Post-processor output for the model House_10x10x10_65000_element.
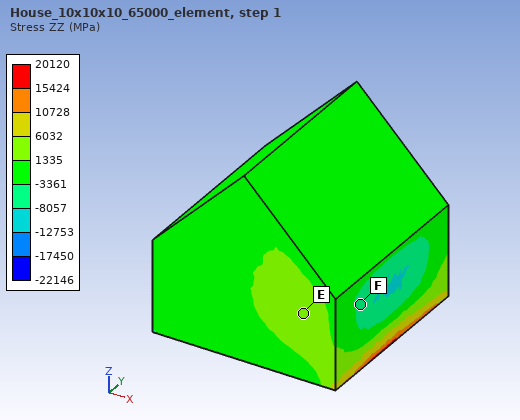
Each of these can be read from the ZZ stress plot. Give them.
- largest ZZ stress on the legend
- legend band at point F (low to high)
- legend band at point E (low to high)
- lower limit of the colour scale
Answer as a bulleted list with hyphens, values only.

- 20120 MPa
- -8057 to -3361 MPa
- 1335 to 6032 MPa
- -22146 MPa
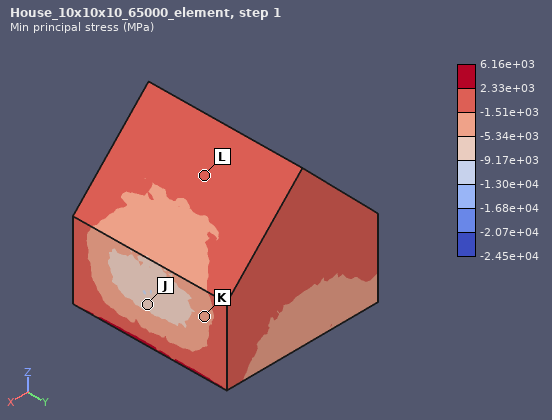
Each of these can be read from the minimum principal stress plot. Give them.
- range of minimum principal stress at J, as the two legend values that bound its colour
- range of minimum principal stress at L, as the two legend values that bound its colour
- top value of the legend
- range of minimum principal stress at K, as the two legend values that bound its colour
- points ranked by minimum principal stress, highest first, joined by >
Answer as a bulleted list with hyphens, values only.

- -9.17e+03 to -5.34e+03 MPa
- -1.51e+03 to 2.33e+03 MPa
- 6.16e+03 MPa
- -5.34e+03 to -1.51e+03 MPa
- L > K > J
